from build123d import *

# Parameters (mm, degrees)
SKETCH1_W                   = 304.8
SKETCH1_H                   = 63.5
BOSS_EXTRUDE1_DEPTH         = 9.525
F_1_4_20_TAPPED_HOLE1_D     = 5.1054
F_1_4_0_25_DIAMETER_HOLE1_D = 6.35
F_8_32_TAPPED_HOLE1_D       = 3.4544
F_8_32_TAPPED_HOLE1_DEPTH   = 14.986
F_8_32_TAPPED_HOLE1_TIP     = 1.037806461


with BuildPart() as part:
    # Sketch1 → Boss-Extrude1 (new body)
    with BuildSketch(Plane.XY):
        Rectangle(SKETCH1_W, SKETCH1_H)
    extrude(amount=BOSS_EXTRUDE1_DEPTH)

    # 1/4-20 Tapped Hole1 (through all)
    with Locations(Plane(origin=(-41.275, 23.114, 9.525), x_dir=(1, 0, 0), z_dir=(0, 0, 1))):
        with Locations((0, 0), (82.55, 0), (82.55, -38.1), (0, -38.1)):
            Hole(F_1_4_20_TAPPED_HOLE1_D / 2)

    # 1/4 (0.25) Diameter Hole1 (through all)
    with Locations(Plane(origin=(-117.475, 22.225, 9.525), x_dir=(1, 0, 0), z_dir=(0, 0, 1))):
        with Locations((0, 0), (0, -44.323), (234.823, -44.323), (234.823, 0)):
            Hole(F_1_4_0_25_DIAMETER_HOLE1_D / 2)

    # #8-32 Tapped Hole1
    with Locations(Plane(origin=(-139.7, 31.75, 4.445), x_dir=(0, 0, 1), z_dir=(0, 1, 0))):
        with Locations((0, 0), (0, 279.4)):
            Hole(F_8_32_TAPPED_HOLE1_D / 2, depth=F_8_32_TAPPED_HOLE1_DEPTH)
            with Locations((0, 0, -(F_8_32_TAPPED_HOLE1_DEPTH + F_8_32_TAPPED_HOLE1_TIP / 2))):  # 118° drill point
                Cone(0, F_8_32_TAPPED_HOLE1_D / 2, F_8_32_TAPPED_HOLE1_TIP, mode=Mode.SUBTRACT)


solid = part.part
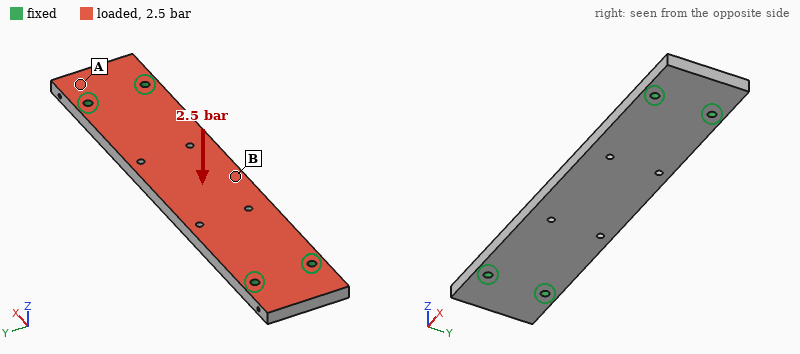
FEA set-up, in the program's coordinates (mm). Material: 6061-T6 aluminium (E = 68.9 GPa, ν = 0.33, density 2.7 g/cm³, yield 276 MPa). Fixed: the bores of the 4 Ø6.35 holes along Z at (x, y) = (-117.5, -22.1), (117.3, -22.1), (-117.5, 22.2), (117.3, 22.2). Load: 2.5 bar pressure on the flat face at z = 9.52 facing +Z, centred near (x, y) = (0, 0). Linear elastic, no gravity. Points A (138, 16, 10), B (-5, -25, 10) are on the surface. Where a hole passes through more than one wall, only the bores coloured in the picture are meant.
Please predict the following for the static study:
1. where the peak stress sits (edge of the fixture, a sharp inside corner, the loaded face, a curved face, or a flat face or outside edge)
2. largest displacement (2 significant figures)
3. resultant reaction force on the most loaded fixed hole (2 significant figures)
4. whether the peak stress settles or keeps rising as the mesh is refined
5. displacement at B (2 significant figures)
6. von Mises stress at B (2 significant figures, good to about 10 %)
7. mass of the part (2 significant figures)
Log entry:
edge of the fixture
0.43 mm
1.2 kN
keeps rising
0.42 mm
38 MPa
490 g
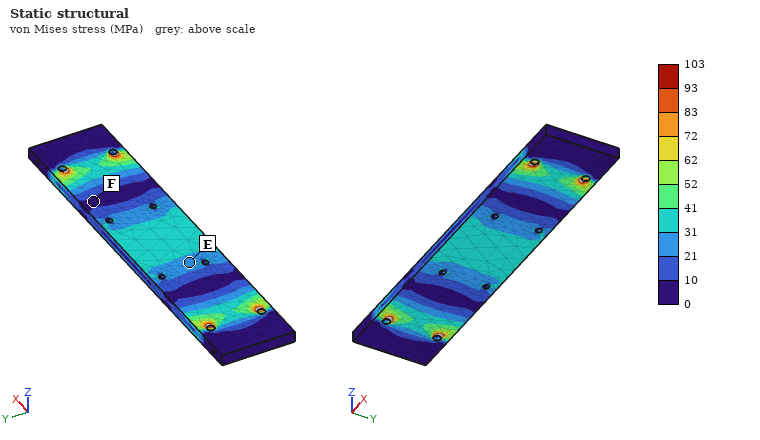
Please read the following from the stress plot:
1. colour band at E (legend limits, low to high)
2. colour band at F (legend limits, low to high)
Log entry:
21 to 31 MPa
0 to 10 MPa
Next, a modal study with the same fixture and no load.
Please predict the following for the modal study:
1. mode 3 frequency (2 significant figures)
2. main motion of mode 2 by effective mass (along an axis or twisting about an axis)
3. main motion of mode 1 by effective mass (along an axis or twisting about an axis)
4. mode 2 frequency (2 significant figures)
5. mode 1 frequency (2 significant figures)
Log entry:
2400 Hz
twisting about X
along Z
2200 Hz
870 Hz
